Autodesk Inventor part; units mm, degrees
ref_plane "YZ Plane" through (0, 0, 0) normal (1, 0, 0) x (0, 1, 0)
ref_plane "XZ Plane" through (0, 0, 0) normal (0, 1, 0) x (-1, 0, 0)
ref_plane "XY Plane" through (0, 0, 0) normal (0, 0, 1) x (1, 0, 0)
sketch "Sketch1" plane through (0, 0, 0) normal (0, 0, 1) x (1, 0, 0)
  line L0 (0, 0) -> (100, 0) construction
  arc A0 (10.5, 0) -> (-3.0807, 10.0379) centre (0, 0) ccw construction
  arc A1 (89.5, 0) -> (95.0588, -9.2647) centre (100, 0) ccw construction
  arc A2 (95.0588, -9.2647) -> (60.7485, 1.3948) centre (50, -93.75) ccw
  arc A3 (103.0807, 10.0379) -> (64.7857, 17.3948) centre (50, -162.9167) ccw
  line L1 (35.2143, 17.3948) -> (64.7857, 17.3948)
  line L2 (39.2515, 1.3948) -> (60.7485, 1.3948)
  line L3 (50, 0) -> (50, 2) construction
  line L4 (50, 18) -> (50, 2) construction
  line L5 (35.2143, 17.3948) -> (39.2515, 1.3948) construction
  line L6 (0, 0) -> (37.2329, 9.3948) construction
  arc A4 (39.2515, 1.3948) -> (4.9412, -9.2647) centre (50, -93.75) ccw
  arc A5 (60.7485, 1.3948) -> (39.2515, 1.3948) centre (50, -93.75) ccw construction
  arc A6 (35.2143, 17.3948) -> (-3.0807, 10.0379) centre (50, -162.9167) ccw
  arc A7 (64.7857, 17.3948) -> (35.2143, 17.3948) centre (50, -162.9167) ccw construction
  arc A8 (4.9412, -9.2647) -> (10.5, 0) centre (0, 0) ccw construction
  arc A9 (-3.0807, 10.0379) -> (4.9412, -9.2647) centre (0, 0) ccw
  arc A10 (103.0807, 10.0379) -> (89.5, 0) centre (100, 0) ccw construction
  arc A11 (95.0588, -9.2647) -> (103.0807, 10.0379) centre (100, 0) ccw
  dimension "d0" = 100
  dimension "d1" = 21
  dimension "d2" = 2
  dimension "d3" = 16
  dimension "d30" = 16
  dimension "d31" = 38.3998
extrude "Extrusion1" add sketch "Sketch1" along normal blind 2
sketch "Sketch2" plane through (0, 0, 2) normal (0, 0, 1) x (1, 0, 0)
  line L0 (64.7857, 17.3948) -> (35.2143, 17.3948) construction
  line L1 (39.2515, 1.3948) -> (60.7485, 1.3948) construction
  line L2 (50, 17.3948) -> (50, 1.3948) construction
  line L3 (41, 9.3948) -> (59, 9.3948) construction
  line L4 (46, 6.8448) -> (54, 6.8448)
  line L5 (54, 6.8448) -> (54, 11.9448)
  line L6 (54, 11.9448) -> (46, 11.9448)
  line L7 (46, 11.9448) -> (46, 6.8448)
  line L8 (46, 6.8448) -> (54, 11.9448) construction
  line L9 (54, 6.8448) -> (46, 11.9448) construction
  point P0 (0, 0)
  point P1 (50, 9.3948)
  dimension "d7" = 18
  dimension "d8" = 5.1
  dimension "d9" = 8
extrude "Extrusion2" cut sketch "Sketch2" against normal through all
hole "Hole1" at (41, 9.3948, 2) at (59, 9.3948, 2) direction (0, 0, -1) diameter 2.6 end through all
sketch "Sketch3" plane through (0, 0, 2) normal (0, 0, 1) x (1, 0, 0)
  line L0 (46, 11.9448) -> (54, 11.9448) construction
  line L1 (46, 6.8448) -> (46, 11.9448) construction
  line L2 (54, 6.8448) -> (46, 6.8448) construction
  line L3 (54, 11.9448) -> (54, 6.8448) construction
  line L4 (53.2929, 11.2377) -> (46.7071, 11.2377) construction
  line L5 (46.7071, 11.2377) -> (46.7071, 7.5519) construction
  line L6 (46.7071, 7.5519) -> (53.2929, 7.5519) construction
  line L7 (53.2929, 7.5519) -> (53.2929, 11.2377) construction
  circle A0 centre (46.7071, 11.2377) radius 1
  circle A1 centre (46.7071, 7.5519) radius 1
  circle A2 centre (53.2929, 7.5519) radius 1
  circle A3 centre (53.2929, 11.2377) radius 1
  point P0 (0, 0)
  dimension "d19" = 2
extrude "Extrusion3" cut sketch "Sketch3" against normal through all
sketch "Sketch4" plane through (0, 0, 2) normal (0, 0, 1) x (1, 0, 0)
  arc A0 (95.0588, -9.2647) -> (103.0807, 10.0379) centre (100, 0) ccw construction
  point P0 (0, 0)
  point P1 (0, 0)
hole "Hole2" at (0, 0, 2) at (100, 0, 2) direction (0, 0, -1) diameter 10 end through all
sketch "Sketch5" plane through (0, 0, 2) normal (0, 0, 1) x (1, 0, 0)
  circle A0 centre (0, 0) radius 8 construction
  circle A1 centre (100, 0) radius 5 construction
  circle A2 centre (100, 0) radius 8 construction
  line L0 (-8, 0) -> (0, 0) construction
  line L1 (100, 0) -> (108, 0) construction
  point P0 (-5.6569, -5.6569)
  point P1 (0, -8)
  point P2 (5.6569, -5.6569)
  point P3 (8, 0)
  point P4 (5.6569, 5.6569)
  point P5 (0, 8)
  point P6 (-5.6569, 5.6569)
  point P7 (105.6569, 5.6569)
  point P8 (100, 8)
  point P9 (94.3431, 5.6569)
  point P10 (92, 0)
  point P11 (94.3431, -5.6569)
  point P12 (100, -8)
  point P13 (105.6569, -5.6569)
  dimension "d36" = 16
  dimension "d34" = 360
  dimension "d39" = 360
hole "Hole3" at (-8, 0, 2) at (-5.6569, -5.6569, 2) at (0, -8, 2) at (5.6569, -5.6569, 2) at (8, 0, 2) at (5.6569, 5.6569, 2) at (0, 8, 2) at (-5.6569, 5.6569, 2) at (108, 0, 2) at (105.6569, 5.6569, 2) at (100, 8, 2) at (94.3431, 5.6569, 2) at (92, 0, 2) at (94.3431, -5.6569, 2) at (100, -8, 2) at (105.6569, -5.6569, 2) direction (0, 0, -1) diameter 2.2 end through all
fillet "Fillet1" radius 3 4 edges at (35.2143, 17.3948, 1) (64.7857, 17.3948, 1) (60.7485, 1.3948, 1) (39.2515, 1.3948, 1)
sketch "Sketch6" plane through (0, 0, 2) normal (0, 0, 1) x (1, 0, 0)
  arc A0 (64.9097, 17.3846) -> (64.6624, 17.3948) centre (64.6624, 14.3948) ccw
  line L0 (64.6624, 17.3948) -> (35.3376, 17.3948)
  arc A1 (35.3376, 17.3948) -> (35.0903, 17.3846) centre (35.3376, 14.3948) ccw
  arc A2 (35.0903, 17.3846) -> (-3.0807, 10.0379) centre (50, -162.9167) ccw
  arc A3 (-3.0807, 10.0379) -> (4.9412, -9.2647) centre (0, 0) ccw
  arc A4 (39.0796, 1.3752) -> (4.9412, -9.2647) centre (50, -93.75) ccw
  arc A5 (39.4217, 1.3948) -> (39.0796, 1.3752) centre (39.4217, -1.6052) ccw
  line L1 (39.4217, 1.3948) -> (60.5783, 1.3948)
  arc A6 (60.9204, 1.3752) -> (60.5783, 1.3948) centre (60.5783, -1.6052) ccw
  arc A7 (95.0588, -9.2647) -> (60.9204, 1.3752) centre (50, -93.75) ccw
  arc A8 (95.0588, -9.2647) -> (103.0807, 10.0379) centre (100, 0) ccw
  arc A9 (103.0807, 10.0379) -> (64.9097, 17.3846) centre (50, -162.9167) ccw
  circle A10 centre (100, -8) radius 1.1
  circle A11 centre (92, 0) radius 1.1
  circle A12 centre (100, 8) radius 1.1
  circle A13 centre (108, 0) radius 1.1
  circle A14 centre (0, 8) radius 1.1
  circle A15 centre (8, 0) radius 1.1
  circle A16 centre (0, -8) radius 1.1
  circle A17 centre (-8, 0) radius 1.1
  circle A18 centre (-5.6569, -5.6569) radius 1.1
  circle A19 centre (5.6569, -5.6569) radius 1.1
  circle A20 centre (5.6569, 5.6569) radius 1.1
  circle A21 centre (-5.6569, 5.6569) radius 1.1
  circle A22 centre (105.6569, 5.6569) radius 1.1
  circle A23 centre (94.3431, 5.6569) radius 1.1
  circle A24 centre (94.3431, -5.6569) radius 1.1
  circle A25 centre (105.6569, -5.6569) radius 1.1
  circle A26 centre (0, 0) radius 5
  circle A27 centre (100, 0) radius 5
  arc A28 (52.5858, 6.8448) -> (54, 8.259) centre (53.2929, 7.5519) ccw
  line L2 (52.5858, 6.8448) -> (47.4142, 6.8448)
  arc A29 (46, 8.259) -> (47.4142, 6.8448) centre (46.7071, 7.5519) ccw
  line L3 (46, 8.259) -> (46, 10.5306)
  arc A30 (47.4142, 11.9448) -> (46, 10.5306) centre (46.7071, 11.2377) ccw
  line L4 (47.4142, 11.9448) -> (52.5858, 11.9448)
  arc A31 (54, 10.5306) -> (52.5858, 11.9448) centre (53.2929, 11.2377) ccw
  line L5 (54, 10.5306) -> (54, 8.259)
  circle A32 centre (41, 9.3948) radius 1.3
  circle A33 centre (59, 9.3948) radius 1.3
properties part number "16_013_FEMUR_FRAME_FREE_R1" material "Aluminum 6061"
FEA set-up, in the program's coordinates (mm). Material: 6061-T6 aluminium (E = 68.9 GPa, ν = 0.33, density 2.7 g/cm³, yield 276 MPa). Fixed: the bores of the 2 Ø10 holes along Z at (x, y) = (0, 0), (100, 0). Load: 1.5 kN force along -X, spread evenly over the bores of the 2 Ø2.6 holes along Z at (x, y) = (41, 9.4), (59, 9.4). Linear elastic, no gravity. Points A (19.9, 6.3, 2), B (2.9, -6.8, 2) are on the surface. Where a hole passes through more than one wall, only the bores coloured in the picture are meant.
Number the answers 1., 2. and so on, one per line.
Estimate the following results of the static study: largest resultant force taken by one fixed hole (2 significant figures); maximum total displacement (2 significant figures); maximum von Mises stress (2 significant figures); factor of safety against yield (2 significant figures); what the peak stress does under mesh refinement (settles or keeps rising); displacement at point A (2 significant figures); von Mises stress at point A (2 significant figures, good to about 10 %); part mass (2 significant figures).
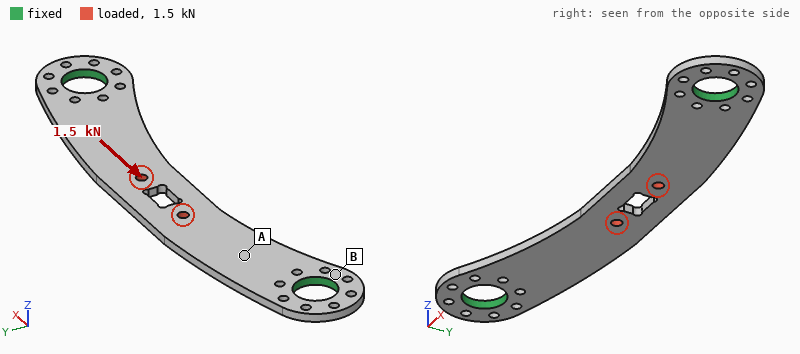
1. 760 N
2. 19 µm
3. 93 MPa
4. 3.0
5. settles
6. 9.3 µm
7. 22 MPa
8. 10 g
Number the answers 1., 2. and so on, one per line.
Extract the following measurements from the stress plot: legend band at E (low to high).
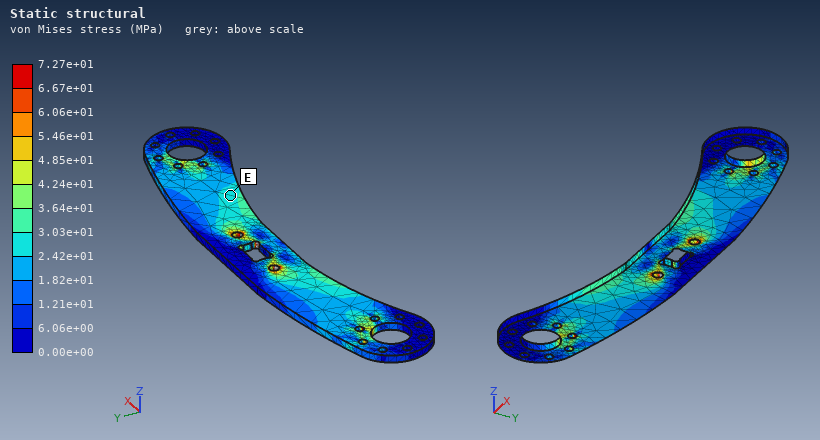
1. 2.42e+01 to 3.03e+01 MPa
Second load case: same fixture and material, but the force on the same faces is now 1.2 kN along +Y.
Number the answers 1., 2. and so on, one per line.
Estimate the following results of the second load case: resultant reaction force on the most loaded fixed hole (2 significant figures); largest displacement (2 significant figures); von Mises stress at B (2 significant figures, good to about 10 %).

1. 960 N
2. 0.11 mm
3. 55 MPa
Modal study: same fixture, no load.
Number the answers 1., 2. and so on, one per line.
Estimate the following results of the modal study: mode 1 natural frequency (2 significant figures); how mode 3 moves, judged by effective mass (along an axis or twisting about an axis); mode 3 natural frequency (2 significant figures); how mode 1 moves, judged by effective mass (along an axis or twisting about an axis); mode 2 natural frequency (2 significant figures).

1. 1200 Hz
2. twisting about X
3. 4200 Hz
4. along Z
5. 3100 Hz
